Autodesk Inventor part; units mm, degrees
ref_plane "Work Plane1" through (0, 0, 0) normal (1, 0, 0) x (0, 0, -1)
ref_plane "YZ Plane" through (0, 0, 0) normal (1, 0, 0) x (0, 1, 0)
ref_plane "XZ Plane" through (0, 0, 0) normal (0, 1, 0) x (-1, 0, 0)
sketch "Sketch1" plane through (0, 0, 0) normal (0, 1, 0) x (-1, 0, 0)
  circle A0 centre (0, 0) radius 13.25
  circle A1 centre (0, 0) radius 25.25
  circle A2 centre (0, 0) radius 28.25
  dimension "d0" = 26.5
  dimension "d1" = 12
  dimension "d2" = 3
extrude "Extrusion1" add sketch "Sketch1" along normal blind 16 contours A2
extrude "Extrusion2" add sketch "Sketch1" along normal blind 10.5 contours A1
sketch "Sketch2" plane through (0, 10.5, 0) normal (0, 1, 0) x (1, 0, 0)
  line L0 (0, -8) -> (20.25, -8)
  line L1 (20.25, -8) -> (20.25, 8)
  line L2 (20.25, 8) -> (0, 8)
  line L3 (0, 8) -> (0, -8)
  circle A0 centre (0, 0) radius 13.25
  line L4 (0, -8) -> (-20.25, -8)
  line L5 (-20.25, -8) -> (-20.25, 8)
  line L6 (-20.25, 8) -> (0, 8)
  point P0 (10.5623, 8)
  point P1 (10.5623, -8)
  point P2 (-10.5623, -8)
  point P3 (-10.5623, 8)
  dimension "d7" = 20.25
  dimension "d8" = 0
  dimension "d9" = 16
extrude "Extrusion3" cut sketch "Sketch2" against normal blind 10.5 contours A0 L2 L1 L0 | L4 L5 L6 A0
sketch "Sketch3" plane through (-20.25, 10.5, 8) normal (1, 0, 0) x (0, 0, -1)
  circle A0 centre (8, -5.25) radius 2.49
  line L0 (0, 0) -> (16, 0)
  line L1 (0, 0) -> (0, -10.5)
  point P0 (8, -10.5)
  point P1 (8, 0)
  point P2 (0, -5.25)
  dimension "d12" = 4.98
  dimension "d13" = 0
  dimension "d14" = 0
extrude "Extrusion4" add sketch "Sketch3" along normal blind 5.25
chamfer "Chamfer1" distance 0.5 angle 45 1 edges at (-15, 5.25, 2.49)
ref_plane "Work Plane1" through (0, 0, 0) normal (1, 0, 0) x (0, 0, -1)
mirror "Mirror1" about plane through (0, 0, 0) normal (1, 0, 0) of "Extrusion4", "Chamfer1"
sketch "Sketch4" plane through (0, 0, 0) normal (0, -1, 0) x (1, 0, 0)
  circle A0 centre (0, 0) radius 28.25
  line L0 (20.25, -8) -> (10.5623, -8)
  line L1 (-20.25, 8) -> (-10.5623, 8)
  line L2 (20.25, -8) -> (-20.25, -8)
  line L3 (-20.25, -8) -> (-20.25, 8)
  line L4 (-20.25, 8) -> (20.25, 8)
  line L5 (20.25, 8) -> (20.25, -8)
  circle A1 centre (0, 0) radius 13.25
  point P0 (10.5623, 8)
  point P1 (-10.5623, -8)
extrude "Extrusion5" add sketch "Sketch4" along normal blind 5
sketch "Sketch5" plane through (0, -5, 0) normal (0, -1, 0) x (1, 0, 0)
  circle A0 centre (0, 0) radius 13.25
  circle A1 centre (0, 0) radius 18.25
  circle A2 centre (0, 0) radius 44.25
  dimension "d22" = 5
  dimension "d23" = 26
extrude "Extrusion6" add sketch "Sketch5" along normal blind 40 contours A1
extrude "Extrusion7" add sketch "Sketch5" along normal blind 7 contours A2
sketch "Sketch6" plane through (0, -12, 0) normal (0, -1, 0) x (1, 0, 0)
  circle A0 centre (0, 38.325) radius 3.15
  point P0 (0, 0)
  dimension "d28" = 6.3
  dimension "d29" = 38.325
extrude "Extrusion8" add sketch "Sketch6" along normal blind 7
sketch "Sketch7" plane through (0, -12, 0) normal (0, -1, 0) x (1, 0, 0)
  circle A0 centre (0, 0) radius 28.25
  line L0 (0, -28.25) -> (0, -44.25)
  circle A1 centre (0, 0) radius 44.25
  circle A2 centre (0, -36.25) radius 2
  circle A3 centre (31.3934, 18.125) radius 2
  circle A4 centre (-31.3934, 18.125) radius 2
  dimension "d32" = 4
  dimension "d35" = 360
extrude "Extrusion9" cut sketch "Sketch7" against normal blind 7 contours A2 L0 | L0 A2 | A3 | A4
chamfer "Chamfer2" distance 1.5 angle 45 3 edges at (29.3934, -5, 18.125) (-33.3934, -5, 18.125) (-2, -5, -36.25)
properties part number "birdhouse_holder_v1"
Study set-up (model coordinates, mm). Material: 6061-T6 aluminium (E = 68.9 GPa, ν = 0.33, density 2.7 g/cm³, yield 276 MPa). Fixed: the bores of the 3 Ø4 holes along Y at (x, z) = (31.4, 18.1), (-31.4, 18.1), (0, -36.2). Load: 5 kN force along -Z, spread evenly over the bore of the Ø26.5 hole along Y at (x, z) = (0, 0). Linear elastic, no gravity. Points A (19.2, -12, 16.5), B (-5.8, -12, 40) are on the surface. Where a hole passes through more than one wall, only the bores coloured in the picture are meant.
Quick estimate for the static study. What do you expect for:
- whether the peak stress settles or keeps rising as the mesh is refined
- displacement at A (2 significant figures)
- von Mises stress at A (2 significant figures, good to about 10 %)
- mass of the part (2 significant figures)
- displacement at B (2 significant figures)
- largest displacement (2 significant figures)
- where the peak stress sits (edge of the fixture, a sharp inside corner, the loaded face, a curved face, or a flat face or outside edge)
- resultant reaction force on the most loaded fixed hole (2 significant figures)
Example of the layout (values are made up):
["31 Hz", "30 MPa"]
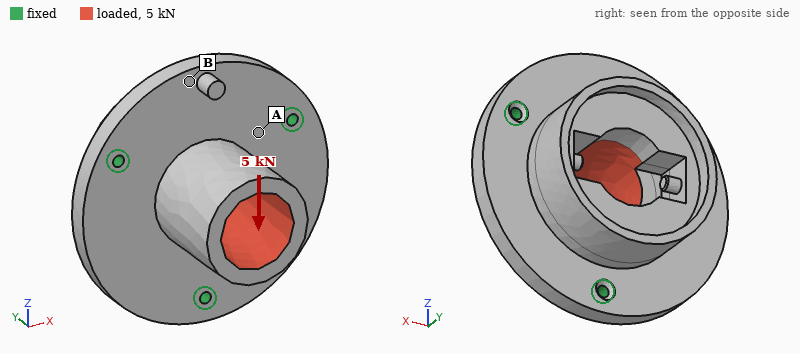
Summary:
["keeps rising", "8.5 µm", "13 MPa", "230 g", "22 µm", "43 µm", "edge of the fixture", "1.9 kN"]
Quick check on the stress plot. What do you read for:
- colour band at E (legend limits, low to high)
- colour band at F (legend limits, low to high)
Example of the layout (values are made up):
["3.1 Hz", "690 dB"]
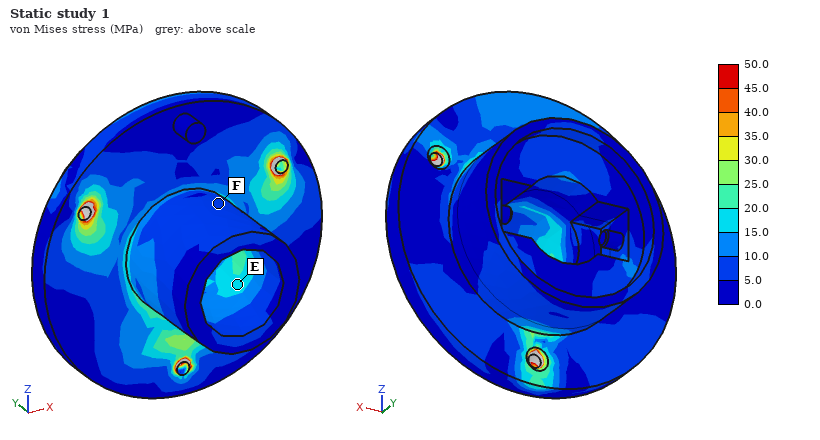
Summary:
["15.0 to 20.0 MPa", "5.0 to 10.0 MPa"]
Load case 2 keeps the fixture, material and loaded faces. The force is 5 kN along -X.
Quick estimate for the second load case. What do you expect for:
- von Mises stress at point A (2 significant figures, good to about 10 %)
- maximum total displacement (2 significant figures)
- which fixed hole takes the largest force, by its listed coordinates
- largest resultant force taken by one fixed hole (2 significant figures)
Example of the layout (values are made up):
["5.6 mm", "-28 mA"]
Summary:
["25 MPa", "43 µm", "(0, -36.2)", "2.1 kN"]
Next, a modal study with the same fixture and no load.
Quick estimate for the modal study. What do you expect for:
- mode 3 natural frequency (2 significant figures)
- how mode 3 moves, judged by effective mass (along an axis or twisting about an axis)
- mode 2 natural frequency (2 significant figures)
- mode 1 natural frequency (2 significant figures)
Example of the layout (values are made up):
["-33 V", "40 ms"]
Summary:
["6200 Hz", "along Y", "5600 Hz", "5500 Hz"]
